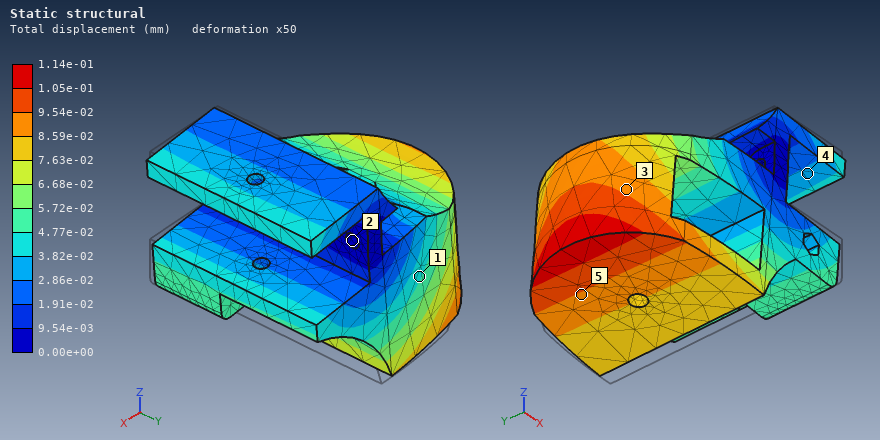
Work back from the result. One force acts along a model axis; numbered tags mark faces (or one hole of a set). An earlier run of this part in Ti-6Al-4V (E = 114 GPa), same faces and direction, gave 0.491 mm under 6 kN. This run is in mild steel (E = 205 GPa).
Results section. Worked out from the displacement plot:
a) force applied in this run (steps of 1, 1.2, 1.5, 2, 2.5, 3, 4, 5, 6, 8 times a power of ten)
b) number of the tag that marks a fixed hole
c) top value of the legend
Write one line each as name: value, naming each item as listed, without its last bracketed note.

force applied in this run: 2.5 kN
number of the tag that marks a fixed hole: 2
top value of the legend: 1.14e-01 mm
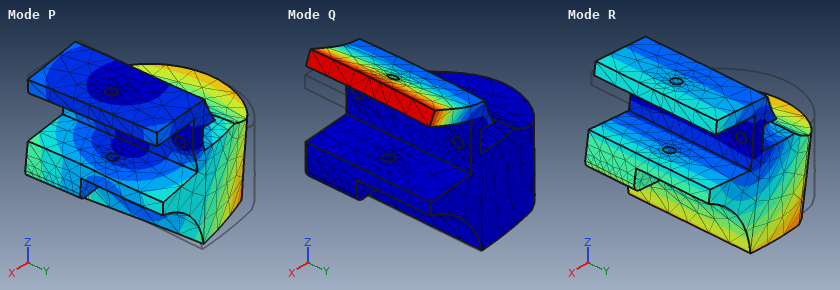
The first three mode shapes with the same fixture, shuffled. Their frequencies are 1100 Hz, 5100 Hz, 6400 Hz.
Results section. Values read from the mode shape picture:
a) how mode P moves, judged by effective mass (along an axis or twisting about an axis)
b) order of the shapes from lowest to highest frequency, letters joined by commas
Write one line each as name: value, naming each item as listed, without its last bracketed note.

how mode P moves, judged by effective mass: along Y
order of the shapes from lowest to highest frequency, letters joined by commas: R, P, Q
